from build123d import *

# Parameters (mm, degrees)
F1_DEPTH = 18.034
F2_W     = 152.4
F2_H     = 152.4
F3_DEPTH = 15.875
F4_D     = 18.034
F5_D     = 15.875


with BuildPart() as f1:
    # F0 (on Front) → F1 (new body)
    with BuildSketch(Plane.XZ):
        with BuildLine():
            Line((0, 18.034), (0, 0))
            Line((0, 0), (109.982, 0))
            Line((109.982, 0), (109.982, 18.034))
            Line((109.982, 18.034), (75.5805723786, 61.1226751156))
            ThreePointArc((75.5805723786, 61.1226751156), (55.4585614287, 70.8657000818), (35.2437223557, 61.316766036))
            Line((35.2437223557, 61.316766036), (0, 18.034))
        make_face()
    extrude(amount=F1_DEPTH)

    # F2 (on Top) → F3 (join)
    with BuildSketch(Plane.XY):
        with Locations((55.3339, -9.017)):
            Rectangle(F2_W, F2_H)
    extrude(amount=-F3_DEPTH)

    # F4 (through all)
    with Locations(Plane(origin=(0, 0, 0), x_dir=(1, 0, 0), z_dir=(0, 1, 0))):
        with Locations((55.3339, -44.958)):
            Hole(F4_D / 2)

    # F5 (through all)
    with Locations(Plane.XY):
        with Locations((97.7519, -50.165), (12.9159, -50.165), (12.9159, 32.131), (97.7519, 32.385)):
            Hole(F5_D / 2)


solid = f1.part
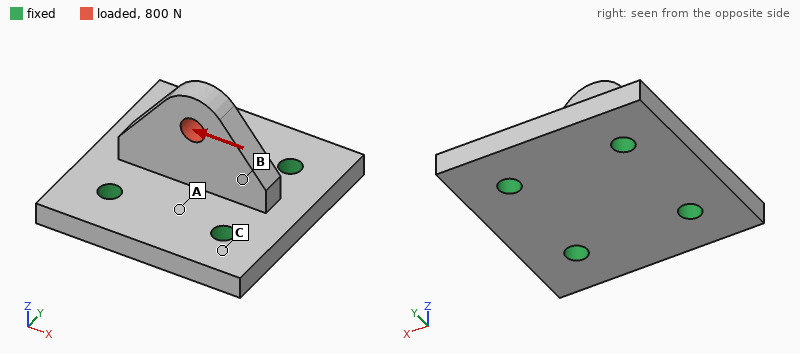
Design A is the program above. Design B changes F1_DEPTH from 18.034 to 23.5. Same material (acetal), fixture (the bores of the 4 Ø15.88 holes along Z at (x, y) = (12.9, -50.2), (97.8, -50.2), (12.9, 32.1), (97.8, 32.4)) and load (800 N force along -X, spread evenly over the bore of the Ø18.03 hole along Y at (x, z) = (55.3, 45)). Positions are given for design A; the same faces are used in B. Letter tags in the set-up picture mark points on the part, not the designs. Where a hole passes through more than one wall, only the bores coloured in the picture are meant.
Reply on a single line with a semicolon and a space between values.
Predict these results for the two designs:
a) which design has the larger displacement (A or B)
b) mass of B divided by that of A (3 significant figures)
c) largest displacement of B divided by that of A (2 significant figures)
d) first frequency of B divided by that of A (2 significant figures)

A; 1.06; 0.85; 1.1
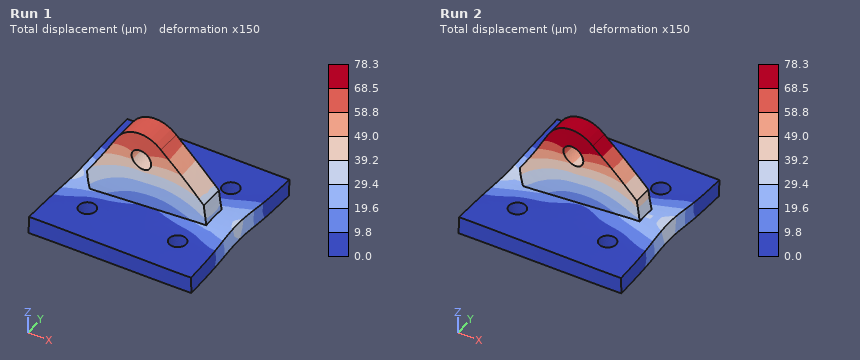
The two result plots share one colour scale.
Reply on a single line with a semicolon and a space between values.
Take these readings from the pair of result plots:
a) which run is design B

Run 1
